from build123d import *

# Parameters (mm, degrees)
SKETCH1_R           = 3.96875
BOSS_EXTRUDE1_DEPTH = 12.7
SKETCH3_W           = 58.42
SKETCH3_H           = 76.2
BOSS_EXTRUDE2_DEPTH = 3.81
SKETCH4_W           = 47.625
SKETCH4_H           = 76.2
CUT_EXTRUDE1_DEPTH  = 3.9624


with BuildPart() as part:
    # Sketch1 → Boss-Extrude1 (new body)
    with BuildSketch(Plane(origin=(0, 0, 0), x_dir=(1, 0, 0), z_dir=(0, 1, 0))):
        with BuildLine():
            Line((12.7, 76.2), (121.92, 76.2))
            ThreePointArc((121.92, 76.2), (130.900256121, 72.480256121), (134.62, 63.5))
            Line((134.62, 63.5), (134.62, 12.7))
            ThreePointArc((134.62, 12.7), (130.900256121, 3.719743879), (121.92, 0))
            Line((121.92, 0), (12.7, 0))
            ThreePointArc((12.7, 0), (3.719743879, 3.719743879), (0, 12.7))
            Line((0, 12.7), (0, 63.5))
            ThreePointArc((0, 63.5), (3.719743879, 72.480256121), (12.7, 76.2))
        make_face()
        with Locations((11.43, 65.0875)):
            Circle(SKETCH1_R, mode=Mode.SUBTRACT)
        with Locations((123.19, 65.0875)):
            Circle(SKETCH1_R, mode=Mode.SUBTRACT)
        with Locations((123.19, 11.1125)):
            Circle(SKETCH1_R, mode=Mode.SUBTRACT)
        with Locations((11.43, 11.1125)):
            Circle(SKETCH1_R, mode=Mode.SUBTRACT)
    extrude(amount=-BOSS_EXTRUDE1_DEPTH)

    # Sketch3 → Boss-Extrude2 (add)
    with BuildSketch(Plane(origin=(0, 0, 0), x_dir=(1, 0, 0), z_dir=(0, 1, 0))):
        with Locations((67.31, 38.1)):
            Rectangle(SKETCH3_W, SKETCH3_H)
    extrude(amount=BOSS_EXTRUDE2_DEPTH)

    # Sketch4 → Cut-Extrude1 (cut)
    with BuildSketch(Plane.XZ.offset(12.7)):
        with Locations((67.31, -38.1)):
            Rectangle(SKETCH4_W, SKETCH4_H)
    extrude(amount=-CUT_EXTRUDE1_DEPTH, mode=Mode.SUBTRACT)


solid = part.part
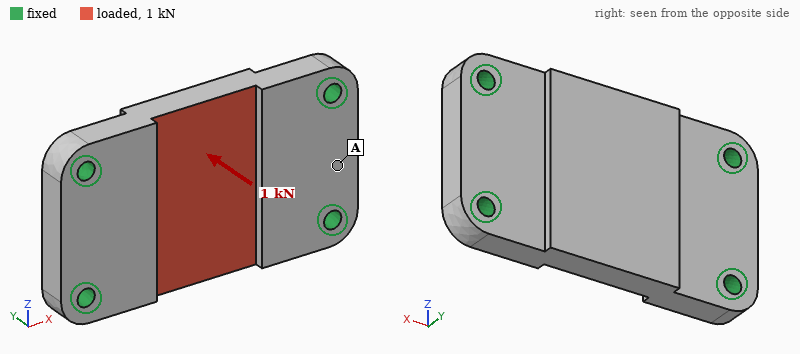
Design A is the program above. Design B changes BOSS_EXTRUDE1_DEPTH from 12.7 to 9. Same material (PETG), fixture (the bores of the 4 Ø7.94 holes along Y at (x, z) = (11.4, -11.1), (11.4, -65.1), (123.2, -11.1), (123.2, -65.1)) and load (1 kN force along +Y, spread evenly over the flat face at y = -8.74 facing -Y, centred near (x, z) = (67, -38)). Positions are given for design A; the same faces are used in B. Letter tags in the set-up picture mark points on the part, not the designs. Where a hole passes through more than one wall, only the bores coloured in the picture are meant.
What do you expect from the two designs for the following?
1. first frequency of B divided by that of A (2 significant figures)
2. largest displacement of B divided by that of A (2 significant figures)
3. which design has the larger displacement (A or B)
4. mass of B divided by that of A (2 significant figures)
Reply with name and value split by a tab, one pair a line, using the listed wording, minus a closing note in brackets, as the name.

first frequency of B divided by that of A	0.78
largest displacement of B divided by that of A	1.7
which design has the larger displacement	B
mass of B divided by that of A	0.82
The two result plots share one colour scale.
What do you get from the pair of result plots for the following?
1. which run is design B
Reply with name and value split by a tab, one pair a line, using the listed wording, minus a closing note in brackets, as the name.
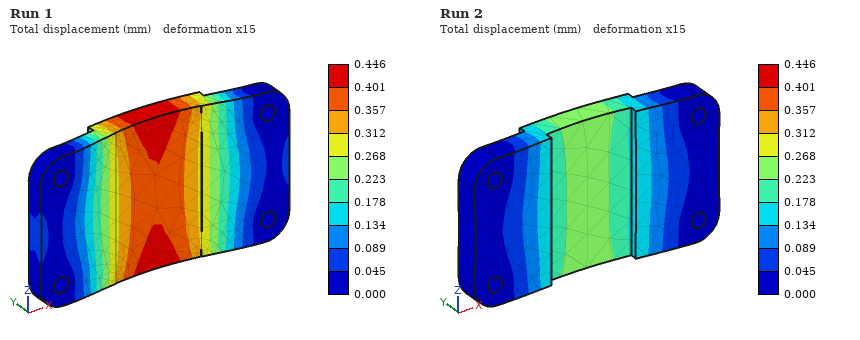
which run is design B	Run 1
